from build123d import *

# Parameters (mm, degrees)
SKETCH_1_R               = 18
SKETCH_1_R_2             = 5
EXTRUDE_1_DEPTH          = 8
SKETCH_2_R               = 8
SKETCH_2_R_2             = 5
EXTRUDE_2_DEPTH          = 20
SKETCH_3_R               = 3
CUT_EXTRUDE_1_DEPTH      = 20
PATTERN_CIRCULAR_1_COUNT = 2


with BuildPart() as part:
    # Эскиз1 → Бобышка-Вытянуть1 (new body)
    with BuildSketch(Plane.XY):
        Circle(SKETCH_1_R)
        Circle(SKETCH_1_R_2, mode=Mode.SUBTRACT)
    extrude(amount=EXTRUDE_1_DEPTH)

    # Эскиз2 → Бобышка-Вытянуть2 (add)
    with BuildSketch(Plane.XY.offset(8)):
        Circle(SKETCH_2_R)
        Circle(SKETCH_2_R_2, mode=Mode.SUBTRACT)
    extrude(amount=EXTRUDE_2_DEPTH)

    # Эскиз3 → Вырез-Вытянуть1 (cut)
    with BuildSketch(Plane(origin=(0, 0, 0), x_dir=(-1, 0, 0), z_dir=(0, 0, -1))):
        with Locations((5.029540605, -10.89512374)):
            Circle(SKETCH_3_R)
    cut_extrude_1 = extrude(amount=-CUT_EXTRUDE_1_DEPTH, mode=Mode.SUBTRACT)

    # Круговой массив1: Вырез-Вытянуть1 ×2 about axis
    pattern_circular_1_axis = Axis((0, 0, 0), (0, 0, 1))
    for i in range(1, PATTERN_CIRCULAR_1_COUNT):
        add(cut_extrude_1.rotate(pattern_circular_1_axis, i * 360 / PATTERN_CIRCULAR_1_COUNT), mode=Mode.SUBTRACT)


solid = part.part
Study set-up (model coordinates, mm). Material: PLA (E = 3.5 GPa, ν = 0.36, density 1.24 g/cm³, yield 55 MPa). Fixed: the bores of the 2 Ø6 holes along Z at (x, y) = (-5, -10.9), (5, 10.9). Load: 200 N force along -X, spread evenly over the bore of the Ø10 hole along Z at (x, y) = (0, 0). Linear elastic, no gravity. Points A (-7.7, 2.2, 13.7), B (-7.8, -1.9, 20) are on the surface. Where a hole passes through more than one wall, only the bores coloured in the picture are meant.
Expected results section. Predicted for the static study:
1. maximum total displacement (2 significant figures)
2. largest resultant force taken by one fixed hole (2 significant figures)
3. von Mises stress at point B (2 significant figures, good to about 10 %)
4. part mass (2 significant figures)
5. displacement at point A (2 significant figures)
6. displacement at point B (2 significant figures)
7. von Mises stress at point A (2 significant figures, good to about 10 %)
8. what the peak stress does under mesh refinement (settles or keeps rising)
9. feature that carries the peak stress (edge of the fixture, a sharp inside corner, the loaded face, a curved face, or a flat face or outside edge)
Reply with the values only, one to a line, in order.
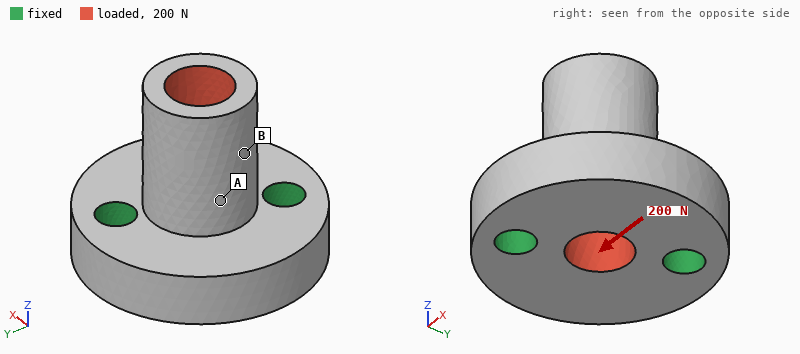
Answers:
71 µm
110 N
0.80 MPa
12 g
32 µm
49 µm
1.9 MPa
keeps rising
edge of the fixture
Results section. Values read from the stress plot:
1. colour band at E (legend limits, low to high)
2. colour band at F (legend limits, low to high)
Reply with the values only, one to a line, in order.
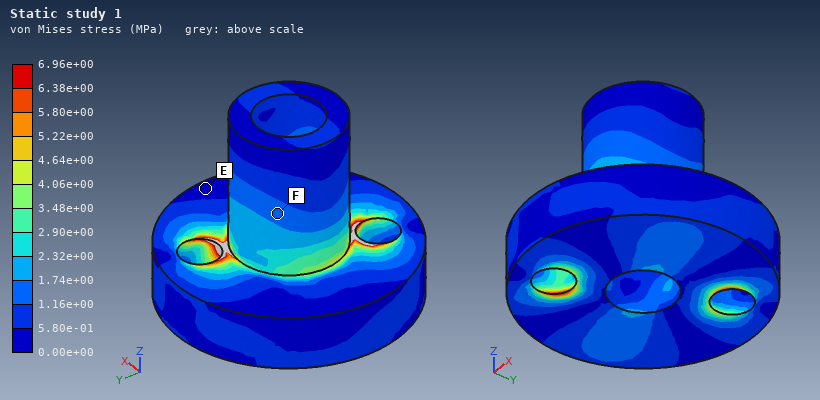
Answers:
0.00e+00 to 5.80e-01 MPa
1.16e+00 to 1.74e+00 MPa
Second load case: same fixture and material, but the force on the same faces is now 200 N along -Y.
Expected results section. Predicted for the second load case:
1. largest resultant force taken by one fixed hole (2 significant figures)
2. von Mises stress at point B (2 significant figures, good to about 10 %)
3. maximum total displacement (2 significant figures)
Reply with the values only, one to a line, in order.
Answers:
130 N
1.3 MPa
52 µm
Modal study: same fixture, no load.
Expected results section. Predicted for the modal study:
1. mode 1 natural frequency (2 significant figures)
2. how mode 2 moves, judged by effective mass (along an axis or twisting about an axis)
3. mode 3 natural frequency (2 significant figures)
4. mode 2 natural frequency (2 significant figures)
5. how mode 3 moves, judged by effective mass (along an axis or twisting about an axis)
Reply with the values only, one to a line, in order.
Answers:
4300 Hz
along Y
8000 Hz
6100 Hz
along Z
